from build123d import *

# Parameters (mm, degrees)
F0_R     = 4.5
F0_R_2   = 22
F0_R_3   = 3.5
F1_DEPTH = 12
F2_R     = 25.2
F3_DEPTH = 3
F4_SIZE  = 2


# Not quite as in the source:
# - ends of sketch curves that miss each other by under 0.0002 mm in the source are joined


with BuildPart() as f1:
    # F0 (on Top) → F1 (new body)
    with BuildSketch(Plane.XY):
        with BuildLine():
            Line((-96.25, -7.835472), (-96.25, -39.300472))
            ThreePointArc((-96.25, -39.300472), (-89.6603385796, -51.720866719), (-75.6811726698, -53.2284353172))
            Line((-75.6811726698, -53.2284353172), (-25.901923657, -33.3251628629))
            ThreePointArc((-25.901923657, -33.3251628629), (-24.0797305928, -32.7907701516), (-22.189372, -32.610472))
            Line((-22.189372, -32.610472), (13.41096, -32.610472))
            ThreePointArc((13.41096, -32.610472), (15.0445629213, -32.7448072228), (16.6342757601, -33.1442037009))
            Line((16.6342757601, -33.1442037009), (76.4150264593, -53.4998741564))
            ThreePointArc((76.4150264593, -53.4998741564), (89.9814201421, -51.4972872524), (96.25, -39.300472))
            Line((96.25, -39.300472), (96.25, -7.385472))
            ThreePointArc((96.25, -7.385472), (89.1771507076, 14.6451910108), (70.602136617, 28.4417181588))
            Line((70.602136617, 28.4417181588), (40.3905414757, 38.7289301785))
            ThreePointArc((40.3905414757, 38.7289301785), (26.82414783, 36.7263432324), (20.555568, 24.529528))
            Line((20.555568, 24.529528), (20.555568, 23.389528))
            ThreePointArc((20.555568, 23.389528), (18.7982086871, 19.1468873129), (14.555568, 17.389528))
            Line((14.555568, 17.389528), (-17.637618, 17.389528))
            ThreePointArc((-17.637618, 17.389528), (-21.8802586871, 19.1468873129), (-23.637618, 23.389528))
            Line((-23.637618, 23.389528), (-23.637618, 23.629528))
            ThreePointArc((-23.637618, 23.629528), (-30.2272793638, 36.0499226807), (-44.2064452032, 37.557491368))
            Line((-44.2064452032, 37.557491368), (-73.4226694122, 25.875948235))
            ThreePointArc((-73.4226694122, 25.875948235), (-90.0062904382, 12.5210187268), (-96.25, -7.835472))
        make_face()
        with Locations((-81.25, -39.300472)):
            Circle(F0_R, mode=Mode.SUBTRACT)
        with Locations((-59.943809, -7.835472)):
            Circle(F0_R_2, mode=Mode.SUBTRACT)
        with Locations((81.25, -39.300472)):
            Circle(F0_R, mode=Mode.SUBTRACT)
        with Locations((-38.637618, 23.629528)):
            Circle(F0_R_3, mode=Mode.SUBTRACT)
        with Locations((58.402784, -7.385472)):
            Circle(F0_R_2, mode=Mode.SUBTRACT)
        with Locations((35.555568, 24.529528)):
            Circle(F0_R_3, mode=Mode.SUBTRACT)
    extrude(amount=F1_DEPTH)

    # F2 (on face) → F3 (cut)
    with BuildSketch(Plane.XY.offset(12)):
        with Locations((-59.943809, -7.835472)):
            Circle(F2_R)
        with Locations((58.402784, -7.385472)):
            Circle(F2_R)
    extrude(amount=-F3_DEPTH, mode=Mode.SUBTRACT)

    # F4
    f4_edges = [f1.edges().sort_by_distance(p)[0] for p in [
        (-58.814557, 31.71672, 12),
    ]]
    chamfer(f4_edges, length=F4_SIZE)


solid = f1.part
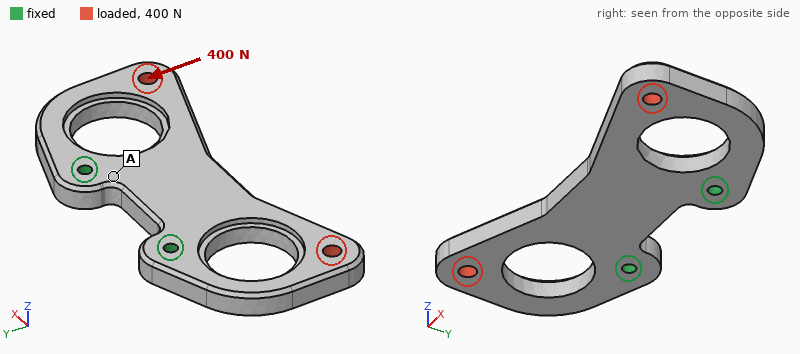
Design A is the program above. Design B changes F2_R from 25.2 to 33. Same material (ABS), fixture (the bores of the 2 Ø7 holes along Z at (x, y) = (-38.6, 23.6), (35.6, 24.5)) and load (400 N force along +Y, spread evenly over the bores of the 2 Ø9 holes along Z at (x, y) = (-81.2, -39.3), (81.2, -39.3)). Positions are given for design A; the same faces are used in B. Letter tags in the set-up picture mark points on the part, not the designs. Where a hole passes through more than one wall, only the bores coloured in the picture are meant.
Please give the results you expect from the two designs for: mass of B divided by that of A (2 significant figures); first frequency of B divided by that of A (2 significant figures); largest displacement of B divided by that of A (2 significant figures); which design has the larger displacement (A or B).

0.93
0.90
1.4
B
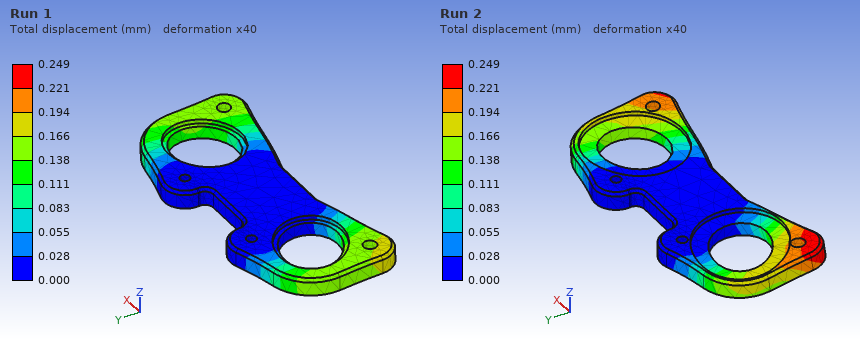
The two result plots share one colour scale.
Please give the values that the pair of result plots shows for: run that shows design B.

Run 2
